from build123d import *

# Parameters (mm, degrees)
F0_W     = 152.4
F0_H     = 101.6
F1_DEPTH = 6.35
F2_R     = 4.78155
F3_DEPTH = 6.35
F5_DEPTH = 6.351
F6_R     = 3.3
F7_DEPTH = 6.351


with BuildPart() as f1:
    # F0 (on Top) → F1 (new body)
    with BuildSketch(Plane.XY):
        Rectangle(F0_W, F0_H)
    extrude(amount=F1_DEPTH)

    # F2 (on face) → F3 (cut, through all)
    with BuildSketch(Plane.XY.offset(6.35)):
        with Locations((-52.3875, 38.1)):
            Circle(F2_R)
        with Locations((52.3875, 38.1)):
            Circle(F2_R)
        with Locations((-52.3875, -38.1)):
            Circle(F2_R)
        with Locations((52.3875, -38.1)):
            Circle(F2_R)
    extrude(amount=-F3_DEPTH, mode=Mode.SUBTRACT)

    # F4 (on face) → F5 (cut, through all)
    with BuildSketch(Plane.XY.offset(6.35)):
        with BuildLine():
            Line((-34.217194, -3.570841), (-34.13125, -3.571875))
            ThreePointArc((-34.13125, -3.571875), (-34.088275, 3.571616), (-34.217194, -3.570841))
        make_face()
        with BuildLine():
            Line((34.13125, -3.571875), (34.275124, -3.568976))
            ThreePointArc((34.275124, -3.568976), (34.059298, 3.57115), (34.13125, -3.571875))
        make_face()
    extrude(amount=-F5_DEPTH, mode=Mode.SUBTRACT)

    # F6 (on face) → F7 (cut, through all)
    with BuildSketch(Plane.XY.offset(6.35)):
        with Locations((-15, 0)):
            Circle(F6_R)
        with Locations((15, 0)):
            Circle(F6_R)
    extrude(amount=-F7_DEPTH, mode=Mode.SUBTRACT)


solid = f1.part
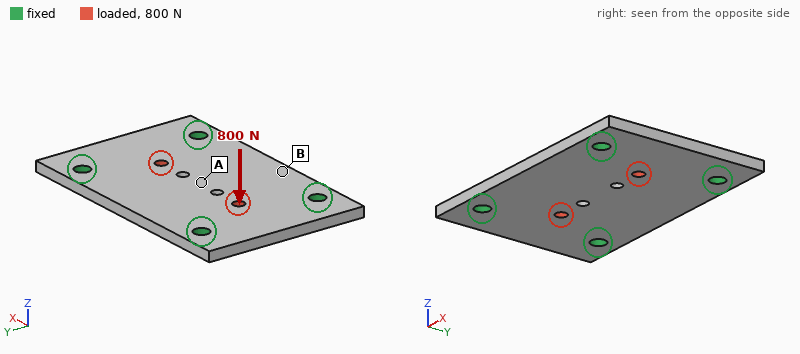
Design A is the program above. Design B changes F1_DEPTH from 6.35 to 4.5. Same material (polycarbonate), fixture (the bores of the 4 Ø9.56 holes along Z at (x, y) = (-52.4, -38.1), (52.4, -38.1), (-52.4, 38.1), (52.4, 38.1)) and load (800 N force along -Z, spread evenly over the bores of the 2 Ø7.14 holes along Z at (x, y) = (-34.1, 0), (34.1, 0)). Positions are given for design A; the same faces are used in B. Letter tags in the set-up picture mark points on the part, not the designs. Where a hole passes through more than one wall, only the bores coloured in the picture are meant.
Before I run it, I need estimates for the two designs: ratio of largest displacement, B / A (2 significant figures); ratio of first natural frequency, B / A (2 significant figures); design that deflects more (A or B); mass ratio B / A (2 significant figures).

2.7
0.73
B
0.71
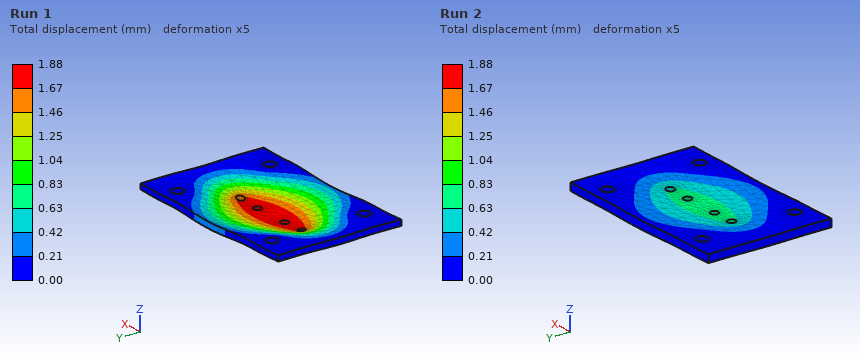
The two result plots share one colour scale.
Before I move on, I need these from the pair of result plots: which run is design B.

Run 1
